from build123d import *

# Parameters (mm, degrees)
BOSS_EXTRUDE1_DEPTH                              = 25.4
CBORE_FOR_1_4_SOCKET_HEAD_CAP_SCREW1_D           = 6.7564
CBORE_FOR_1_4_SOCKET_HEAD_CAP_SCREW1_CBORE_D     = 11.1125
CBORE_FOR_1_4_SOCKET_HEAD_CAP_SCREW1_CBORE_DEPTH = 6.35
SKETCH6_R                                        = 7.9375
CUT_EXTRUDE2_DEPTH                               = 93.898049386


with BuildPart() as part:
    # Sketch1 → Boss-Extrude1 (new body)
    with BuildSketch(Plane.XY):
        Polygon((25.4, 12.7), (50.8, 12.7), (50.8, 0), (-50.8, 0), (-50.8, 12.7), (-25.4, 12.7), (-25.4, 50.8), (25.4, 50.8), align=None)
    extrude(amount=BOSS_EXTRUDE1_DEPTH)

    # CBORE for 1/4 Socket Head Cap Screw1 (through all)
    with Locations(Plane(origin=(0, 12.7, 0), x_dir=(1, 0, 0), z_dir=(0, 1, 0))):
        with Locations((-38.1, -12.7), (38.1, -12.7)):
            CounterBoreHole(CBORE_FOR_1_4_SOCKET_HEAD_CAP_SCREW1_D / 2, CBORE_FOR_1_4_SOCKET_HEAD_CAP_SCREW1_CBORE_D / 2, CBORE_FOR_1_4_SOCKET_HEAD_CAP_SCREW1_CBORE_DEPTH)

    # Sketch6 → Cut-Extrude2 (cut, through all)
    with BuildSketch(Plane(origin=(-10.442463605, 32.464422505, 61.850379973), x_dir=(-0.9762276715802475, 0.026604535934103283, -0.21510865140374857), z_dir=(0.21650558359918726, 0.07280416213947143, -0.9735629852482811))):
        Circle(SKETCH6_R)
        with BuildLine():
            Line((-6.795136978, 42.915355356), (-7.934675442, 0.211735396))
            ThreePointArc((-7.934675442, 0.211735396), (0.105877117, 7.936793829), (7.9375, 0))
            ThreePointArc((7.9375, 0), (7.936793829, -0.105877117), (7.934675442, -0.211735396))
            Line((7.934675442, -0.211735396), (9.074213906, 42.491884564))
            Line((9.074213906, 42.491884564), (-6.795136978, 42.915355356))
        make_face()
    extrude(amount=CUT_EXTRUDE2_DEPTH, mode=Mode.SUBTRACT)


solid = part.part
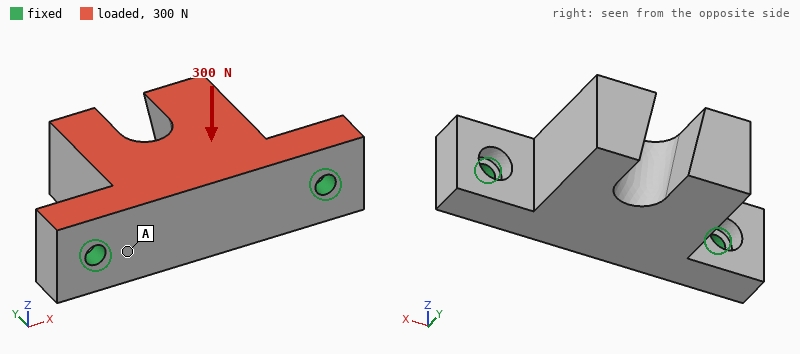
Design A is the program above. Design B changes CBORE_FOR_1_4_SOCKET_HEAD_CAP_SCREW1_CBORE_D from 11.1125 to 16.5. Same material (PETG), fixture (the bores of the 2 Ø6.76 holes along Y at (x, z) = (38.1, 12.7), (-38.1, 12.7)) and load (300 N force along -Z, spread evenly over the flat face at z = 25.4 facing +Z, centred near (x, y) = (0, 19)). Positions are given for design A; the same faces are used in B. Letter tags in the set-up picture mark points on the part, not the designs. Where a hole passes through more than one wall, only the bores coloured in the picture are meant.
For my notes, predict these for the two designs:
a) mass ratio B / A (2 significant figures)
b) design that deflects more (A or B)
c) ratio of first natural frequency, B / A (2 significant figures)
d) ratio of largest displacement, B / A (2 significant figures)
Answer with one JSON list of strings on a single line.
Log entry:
["0.98", "B", "0.93", "1.1"]
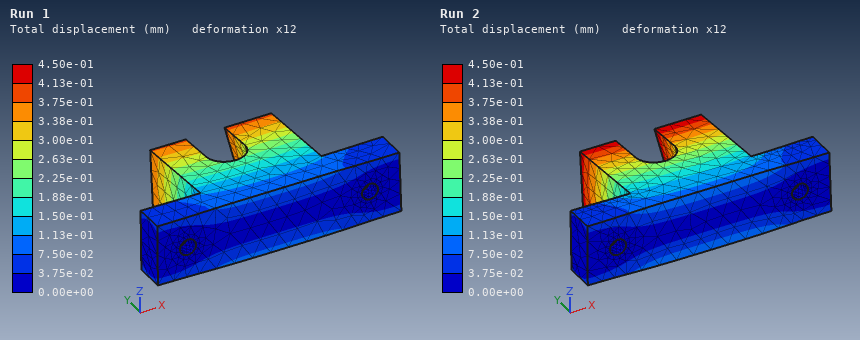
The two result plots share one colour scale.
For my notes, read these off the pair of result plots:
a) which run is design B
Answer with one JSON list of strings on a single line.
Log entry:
["Run 2"]
